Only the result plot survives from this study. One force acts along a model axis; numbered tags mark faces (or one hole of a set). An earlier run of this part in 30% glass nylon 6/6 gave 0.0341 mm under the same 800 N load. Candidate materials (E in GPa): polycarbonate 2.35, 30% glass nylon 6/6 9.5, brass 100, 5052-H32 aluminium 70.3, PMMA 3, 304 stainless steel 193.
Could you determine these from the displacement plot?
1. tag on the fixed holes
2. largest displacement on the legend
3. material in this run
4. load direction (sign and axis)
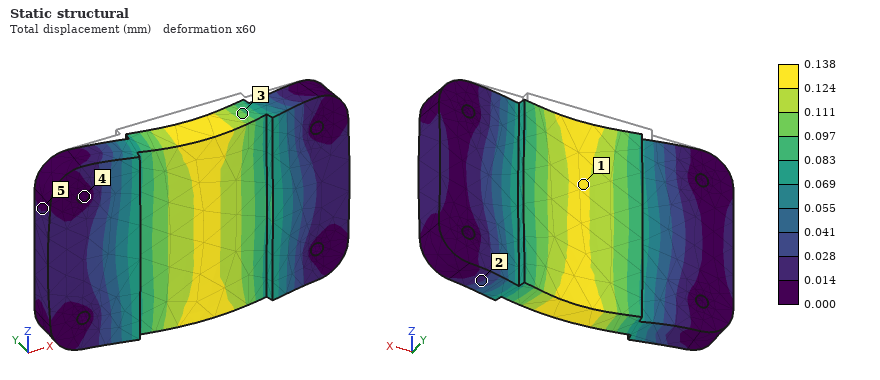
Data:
4
0.138 mm
polycarbonate
-Y
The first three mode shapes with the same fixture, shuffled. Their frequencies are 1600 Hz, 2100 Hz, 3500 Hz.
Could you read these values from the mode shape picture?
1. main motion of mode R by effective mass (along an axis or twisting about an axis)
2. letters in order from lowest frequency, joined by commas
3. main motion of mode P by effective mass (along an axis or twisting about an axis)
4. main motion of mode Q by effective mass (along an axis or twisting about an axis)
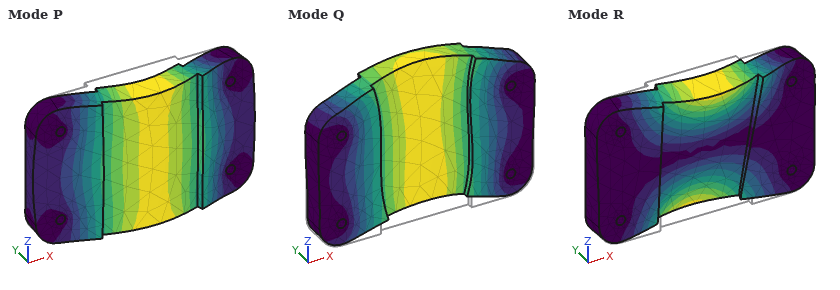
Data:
twisting about X
P, R, Q
along Y
along Z
